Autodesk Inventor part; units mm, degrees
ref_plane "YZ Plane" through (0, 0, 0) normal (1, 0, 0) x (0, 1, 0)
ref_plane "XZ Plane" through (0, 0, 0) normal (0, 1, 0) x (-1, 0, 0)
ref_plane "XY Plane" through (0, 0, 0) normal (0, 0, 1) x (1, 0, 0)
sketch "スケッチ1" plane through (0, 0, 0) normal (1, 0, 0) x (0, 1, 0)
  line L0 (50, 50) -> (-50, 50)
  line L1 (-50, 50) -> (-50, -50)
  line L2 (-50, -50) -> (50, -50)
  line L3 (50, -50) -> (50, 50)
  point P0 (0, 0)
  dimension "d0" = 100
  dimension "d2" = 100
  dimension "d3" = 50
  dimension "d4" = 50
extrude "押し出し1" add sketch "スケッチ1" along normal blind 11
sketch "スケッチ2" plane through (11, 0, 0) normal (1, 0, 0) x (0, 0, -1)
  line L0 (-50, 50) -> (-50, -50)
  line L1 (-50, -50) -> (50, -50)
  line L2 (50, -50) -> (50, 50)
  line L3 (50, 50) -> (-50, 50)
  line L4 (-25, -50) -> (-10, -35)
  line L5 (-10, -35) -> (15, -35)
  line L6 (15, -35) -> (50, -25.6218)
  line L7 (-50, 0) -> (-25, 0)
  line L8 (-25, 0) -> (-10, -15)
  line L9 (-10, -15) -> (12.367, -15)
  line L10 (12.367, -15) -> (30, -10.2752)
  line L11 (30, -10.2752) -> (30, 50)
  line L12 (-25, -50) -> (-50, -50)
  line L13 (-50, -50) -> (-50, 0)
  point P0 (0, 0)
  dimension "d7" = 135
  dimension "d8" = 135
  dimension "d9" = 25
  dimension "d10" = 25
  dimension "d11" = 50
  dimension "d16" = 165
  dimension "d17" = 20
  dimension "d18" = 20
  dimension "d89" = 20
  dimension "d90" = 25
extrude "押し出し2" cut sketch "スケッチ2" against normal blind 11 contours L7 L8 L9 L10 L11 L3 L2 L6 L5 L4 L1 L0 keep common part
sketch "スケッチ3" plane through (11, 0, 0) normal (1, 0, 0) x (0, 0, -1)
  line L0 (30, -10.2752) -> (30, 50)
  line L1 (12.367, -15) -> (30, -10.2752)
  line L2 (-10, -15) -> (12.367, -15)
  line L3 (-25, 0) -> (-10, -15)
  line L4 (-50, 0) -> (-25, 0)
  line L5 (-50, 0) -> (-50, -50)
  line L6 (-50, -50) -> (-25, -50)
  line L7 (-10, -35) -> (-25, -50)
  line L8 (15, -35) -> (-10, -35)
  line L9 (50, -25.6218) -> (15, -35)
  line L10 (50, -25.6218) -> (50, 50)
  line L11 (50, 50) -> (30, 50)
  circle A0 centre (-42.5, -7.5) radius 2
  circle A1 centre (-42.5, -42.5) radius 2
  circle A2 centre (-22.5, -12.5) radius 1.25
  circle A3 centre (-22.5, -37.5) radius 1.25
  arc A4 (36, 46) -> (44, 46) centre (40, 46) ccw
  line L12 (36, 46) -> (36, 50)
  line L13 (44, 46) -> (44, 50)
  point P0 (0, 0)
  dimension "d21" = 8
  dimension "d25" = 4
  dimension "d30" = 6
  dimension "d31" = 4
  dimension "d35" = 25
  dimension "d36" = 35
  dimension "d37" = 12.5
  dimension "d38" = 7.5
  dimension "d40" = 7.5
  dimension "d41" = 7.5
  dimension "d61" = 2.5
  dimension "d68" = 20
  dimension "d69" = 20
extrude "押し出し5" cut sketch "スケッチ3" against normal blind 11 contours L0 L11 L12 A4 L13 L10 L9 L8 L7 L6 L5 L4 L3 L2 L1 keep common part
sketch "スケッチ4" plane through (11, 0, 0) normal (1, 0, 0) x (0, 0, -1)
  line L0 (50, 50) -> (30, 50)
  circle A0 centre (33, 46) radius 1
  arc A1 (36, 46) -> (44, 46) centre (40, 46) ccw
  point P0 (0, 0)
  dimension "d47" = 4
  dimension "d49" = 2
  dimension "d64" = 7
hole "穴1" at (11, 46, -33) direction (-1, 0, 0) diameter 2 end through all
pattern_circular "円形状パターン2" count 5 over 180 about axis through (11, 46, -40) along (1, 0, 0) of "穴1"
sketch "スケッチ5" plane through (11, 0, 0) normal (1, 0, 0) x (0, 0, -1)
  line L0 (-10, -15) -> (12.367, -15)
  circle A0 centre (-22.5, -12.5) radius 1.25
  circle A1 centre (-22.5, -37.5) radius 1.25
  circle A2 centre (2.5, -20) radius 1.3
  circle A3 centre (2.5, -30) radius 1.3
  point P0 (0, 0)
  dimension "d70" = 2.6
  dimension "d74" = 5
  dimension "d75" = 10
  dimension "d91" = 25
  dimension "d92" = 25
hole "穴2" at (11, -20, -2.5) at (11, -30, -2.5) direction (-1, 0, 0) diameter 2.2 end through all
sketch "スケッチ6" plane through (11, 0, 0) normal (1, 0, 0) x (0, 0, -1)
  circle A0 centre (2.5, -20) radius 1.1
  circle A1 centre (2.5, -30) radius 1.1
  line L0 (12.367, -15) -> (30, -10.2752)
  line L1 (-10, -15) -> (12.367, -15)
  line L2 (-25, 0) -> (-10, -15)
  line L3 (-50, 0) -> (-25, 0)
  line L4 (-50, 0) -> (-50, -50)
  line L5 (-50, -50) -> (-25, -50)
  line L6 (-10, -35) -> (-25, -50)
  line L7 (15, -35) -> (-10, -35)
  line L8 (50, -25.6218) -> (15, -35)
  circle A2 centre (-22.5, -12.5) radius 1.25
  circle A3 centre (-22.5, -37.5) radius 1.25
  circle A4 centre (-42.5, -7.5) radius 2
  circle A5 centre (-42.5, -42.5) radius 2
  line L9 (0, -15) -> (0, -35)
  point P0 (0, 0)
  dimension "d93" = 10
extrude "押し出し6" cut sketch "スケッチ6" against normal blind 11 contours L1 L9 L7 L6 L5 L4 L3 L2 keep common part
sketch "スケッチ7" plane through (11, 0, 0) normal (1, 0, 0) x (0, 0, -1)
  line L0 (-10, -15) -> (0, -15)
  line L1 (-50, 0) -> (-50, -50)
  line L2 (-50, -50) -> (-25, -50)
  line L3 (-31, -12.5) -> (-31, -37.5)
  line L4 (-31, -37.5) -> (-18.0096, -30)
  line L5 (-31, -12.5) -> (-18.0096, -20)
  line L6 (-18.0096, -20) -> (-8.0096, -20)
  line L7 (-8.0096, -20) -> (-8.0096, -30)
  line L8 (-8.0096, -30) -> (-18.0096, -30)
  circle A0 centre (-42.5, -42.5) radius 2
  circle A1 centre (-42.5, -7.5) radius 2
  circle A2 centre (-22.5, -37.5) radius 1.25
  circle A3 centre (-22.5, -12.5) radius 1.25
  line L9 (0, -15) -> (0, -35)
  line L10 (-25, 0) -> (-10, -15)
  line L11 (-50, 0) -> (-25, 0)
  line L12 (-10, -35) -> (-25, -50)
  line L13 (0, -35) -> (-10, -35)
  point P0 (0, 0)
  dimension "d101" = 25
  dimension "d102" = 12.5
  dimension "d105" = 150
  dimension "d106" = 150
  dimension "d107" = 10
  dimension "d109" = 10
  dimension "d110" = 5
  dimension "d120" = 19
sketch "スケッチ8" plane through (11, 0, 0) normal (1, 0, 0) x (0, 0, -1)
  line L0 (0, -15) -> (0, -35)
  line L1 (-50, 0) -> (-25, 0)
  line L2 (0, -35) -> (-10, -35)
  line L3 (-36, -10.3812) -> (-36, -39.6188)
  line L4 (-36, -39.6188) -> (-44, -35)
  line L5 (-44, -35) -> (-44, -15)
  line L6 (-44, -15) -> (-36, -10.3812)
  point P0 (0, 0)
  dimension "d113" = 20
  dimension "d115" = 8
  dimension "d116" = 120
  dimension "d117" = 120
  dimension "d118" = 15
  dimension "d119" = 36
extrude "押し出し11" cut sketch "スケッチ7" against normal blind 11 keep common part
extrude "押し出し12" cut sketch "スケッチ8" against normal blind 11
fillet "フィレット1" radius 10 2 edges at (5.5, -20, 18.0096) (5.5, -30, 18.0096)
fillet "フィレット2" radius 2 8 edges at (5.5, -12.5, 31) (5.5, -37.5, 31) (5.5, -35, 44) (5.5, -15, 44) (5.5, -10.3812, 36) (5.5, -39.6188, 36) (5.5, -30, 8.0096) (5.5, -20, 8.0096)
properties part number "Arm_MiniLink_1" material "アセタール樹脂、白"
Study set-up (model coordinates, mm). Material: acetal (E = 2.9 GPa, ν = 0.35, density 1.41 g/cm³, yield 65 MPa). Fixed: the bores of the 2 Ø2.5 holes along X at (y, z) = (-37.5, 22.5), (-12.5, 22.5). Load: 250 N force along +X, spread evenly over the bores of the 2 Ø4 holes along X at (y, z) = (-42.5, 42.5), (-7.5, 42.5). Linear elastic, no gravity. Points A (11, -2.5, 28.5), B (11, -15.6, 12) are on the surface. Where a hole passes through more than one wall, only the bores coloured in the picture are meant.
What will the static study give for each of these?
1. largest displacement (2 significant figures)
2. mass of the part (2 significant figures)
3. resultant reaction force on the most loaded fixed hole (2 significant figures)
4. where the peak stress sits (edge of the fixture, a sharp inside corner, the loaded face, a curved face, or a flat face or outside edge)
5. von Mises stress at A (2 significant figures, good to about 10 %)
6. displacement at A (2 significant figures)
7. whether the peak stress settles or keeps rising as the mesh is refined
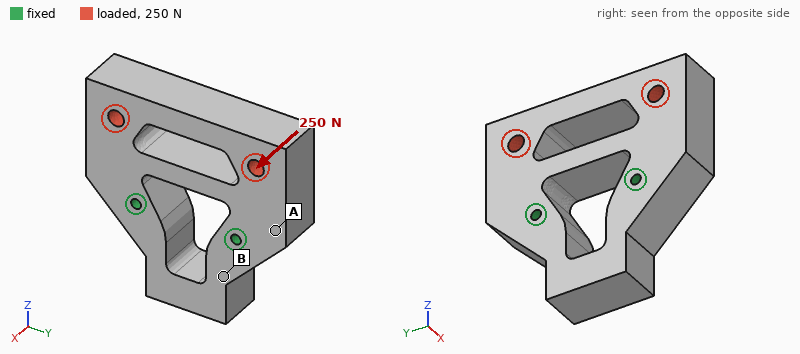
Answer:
0.21 mm
22 g
130 N
edge of the fixture
3.8 MPa
0.046 mm
keeps rising
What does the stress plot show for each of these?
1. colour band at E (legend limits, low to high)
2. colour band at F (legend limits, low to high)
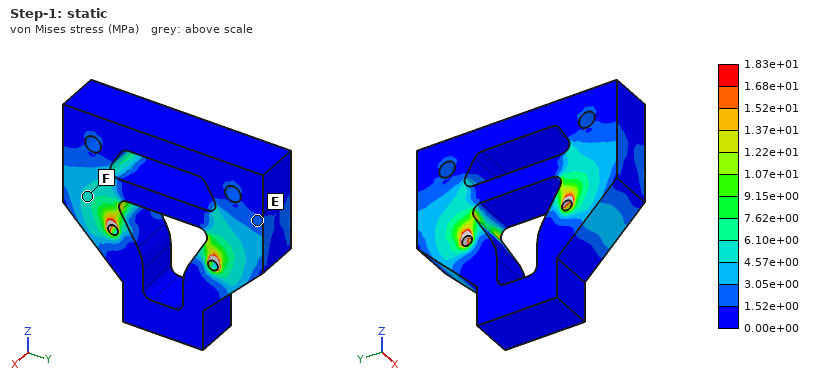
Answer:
1.52e+00 to 3.05e+00 MPa
4.57e+00 to 6.10e+00 MPa
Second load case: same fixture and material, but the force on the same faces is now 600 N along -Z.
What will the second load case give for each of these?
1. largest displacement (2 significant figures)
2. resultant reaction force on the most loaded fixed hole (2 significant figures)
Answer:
29 µm
300 N
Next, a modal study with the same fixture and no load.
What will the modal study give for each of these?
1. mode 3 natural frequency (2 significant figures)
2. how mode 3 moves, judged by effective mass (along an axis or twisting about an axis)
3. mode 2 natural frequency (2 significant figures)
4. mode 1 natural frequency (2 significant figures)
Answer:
3000 Hz
twisting about Z
2100 Hz
2000 Hz
